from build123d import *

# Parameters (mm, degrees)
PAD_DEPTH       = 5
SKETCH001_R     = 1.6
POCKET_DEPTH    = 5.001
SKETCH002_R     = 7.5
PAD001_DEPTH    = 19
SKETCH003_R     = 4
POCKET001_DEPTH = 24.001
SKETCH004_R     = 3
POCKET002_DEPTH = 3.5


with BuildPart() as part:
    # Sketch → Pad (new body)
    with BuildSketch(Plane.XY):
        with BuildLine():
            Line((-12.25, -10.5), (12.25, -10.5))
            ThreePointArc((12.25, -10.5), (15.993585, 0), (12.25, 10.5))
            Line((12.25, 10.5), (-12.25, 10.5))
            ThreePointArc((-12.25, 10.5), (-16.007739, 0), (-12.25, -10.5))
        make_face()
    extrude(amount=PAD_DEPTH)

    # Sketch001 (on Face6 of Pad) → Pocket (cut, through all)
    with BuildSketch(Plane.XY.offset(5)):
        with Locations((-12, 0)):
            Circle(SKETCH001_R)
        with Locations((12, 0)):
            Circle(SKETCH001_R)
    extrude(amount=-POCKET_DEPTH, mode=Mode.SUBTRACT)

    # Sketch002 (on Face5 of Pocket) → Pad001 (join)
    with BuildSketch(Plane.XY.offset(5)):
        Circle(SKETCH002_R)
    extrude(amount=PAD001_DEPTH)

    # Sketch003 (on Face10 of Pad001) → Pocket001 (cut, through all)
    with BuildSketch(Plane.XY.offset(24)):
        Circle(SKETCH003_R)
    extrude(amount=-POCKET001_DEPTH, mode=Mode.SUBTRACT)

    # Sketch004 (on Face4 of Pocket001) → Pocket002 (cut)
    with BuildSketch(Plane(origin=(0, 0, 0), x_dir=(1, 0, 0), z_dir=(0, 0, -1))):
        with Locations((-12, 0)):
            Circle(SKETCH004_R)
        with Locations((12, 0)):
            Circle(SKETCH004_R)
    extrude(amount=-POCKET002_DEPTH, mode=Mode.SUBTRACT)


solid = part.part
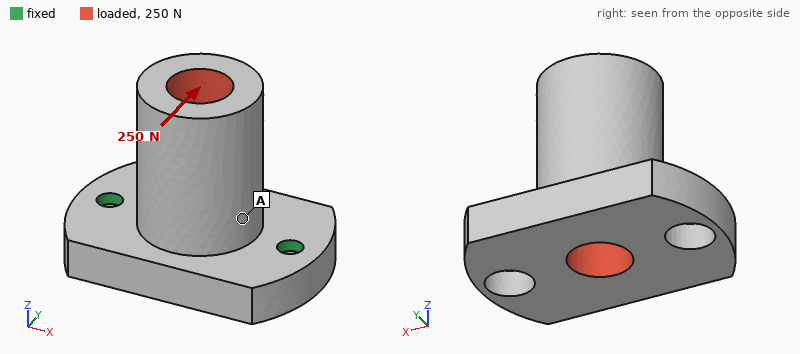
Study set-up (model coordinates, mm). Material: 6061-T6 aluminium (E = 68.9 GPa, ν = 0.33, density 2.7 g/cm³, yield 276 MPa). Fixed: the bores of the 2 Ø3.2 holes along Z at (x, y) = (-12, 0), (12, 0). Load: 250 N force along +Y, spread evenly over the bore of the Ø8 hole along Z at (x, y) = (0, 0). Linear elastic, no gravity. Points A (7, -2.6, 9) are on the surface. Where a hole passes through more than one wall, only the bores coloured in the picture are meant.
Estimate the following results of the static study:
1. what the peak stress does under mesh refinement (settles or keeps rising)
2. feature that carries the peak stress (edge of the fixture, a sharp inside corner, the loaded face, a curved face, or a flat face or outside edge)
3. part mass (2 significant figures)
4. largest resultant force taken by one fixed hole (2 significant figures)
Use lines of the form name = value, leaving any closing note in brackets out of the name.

what the peak stress does under mesh refinement = keeps rising
feature that carries the peak stress = edge of the fixture
part mass = 14 g
largest resultant force taken by one fixed hole = 130 N
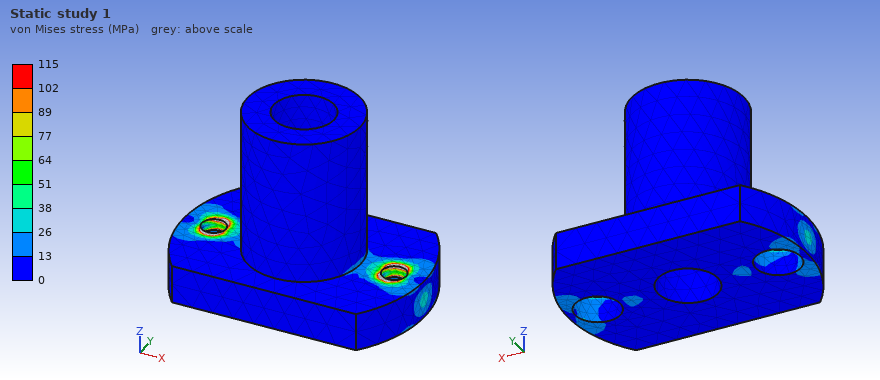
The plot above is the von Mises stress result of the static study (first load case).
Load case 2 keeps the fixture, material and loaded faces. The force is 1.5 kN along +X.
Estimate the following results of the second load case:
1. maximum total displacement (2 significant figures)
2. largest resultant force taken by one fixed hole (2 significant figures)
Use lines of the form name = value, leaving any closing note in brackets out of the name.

maximum total displacement = 39 µm
largest resultant force taken by one fixed hole = 920 N
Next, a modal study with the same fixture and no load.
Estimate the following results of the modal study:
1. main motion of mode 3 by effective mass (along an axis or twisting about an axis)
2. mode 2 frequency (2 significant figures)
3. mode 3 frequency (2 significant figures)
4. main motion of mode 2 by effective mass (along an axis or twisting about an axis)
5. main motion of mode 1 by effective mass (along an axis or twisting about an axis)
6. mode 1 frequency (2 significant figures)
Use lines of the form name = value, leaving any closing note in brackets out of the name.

main motion of mode 3 by effective mass = along Z
mode 2 frequency = 13 kHz
mode 3 frequency = 15 kHz
main motion of mode 2 by effective mass = along X
main motion of mode 1 by effective mass = along Y
mode 1 frequency = 4200 Hz
